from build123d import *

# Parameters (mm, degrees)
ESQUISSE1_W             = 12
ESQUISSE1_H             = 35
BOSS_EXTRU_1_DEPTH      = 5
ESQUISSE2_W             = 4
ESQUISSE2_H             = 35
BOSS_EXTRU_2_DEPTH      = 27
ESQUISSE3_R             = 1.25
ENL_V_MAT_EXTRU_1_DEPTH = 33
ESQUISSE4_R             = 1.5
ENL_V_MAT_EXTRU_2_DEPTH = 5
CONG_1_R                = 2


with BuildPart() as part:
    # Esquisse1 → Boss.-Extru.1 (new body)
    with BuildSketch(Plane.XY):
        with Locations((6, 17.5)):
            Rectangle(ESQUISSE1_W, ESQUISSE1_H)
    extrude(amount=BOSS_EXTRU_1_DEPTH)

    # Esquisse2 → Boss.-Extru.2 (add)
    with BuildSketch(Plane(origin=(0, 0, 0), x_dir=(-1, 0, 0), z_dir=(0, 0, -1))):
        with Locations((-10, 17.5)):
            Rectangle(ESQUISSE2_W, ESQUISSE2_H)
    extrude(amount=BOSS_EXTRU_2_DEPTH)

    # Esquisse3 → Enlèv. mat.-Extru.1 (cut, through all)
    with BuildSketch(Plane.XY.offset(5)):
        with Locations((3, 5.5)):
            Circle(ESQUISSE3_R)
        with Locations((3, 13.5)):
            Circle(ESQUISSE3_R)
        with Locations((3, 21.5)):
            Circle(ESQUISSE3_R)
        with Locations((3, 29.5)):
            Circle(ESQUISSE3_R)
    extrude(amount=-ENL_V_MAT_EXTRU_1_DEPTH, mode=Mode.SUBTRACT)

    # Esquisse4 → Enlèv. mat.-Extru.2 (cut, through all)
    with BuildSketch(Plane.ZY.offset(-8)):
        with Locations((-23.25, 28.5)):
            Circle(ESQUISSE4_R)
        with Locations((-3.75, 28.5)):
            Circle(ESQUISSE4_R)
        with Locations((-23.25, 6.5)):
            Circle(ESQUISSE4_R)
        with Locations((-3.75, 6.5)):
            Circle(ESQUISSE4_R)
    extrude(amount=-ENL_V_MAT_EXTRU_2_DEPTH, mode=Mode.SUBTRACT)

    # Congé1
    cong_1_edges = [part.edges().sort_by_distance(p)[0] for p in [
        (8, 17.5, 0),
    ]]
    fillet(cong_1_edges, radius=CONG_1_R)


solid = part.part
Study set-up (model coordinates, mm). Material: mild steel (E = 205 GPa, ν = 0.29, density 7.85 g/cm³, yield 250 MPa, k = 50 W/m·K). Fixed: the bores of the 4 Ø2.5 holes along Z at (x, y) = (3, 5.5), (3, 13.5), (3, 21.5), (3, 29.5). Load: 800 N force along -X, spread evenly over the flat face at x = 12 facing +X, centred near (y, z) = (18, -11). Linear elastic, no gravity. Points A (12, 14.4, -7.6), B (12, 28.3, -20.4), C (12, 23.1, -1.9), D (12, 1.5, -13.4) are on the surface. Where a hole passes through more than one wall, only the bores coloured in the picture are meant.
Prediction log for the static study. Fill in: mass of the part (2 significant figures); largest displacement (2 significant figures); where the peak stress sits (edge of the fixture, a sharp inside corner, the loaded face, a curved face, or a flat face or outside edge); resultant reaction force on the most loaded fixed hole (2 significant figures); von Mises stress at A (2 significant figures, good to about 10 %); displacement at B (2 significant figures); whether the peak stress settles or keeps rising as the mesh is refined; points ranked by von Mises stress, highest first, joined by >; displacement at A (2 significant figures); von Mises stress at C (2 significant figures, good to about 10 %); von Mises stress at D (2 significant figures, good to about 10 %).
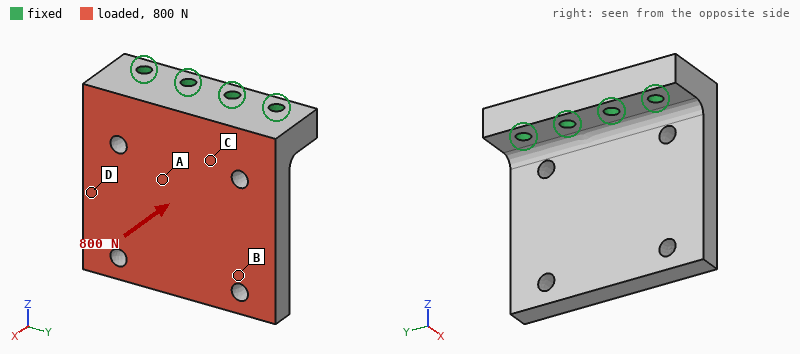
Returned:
45 g
74 µm
edge of the fixture
230 N
49 MPa
53 µm
keeps rising
C > A > D > B
18 µm
82 MPa
26 MPa
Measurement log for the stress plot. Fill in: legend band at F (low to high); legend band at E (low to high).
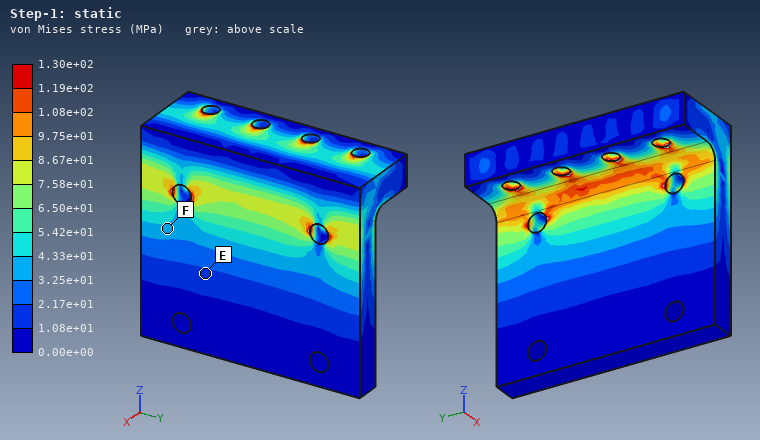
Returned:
3.25e+01 to 4.33e+01 MPa
1.08e+01 to 2.17e+01 MPa
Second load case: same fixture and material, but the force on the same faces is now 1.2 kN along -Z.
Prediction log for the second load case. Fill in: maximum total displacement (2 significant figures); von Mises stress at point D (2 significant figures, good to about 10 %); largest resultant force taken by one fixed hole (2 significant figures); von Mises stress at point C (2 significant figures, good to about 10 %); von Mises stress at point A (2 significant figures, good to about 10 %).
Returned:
33 µm
15 MPa
310 N
28 MPa
21 MPa
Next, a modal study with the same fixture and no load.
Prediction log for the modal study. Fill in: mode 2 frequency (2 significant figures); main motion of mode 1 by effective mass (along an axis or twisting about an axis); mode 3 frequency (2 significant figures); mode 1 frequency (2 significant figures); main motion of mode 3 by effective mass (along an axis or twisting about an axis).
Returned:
7500 Hz
along X
11 kHz
3500 Hz
along Y
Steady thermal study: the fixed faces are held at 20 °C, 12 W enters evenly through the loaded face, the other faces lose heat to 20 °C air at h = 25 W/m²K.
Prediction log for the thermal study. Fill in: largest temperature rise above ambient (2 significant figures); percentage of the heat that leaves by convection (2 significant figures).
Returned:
28 K
7.0 %
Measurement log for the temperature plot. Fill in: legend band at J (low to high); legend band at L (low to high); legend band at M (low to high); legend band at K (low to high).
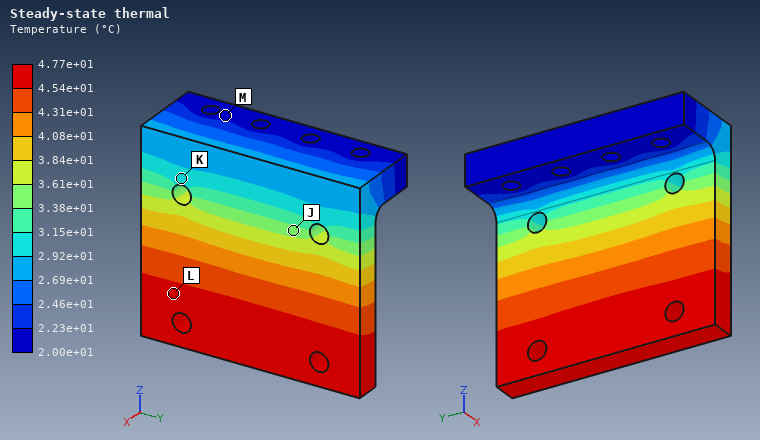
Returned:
3.38e+01 to 3.61e+01 °C
4.54e+01 to 4.77e+01 °C
2.00e+01 to 2.23e+01 °C
2.92e+01 to 3.15e+01 °C
